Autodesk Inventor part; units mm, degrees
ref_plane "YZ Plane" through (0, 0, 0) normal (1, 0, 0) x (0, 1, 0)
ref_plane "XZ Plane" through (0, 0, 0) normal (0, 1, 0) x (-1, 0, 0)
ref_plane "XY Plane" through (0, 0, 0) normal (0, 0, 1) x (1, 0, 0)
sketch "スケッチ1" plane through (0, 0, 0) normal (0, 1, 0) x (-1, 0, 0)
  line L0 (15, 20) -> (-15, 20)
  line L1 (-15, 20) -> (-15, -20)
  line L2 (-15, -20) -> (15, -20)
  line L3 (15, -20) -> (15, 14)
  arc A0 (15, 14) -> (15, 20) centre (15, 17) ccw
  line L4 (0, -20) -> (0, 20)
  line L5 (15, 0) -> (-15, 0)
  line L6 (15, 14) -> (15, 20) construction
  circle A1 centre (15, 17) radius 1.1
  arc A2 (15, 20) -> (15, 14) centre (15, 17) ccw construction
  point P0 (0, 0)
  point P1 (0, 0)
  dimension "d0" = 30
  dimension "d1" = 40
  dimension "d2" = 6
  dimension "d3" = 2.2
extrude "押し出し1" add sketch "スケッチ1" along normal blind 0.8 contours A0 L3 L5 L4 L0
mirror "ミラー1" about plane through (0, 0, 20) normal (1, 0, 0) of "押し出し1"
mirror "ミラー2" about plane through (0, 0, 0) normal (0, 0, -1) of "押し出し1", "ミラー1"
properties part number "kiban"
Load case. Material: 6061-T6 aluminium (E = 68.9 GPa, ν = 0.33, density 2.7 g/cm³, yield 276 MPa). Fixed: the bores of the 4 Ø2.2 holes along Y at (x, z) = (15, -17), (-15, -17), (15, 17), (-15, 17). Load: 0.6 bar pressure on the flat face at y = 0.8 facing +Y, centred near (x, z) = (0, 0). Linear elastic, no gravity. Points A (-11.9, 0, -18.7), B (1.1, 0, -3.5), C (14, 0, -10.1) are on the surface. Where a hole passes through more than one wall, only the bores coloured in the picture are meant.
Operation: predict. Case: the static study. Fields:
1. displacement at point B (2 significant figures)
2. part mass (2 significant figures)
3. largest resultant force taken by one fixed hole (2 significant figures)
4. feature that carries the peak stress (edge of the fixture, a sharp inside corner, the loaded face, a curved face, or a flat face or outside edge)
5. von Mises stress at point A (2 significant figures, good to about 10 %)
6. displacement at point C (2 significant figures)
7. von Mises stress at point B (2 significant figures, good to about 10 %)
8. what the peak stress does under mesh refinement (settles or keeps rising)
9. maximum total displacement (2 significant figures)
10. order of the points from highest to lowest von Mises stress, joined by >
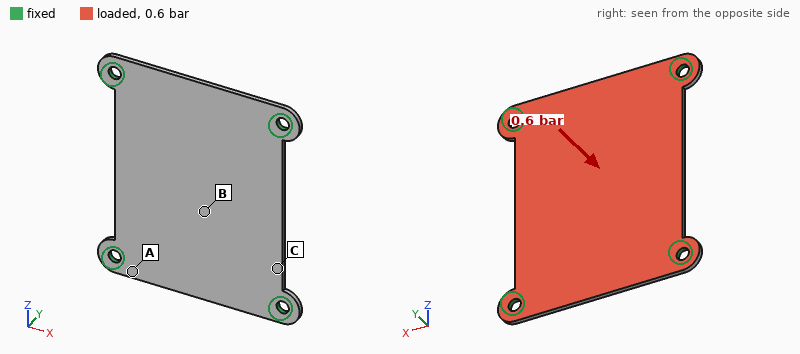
0.14 mm
2.7 g
19 N
edge of the fixture
49 MPa
0.043 mm
30 MPa
keeps rising
0.14 mm
A > B > C
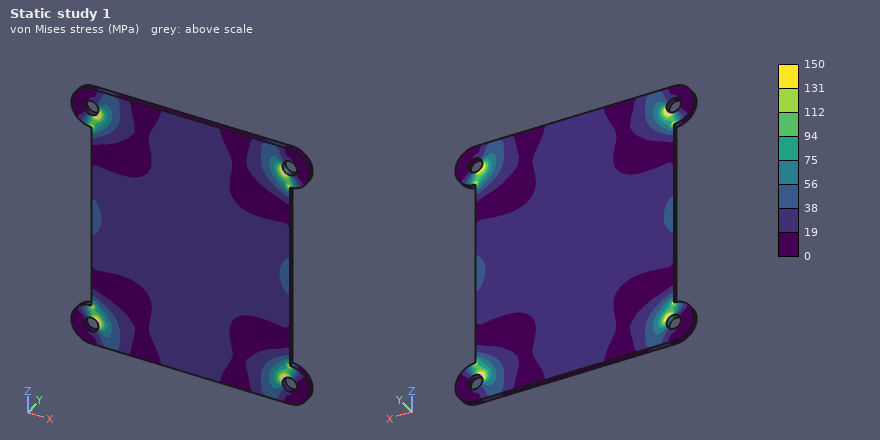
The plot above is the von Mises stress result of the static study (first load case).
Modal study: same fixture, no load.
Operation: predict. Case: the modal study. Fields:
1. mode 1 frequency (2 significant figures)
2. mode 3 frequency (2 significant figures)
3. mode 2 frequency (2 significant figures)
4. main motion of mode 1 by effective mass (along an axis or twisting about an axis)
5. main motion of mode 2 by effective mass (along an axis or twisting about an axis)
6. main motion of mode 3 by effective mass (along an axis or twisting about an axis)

2600 Hz
5100 Hz
4600 Hz
along Y
twisting about Z
twisting about X
